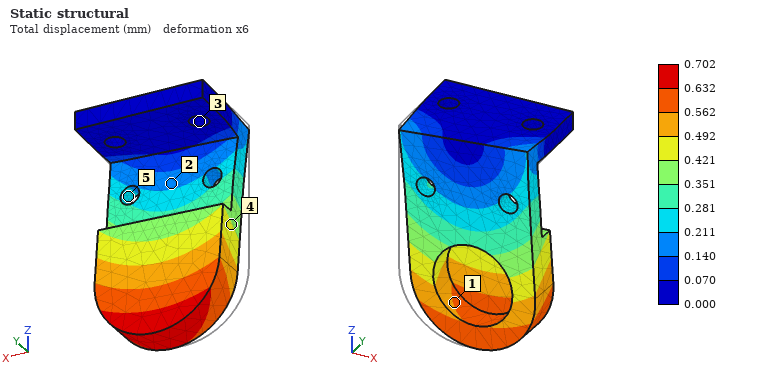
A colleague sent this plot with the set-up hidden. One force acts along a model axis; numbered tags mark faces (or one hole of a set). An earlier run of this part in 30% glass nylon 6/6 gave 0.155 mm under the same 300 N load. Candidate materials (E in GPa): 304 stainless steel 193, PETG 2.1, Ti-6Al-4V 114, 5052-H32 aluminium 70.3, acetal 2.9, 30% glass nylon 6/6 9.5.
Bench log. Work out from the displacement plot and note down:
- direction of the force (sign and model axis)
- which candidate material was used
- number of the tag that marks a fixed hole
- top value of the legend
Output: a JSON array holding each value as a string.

["+X", "PETG", "3", "0.702 mm"]
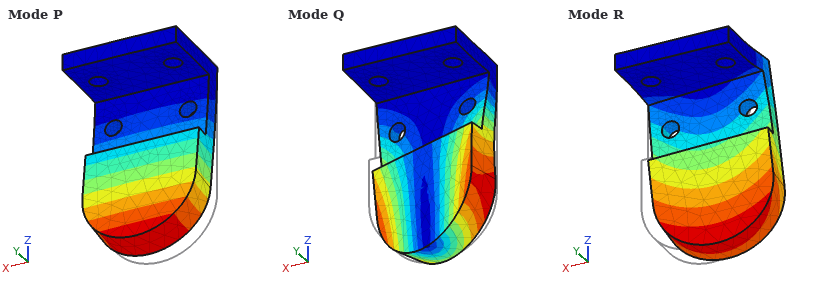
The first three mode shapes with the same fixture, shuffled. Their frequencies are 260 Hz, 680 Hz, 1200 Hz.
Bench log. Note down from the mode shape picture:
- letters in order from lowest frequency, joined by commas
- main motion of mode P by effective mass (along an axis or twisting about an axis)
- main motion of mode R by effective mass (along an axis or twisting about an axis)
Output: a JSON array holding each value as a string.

["P, R, Q", "along Y", "along X"]
